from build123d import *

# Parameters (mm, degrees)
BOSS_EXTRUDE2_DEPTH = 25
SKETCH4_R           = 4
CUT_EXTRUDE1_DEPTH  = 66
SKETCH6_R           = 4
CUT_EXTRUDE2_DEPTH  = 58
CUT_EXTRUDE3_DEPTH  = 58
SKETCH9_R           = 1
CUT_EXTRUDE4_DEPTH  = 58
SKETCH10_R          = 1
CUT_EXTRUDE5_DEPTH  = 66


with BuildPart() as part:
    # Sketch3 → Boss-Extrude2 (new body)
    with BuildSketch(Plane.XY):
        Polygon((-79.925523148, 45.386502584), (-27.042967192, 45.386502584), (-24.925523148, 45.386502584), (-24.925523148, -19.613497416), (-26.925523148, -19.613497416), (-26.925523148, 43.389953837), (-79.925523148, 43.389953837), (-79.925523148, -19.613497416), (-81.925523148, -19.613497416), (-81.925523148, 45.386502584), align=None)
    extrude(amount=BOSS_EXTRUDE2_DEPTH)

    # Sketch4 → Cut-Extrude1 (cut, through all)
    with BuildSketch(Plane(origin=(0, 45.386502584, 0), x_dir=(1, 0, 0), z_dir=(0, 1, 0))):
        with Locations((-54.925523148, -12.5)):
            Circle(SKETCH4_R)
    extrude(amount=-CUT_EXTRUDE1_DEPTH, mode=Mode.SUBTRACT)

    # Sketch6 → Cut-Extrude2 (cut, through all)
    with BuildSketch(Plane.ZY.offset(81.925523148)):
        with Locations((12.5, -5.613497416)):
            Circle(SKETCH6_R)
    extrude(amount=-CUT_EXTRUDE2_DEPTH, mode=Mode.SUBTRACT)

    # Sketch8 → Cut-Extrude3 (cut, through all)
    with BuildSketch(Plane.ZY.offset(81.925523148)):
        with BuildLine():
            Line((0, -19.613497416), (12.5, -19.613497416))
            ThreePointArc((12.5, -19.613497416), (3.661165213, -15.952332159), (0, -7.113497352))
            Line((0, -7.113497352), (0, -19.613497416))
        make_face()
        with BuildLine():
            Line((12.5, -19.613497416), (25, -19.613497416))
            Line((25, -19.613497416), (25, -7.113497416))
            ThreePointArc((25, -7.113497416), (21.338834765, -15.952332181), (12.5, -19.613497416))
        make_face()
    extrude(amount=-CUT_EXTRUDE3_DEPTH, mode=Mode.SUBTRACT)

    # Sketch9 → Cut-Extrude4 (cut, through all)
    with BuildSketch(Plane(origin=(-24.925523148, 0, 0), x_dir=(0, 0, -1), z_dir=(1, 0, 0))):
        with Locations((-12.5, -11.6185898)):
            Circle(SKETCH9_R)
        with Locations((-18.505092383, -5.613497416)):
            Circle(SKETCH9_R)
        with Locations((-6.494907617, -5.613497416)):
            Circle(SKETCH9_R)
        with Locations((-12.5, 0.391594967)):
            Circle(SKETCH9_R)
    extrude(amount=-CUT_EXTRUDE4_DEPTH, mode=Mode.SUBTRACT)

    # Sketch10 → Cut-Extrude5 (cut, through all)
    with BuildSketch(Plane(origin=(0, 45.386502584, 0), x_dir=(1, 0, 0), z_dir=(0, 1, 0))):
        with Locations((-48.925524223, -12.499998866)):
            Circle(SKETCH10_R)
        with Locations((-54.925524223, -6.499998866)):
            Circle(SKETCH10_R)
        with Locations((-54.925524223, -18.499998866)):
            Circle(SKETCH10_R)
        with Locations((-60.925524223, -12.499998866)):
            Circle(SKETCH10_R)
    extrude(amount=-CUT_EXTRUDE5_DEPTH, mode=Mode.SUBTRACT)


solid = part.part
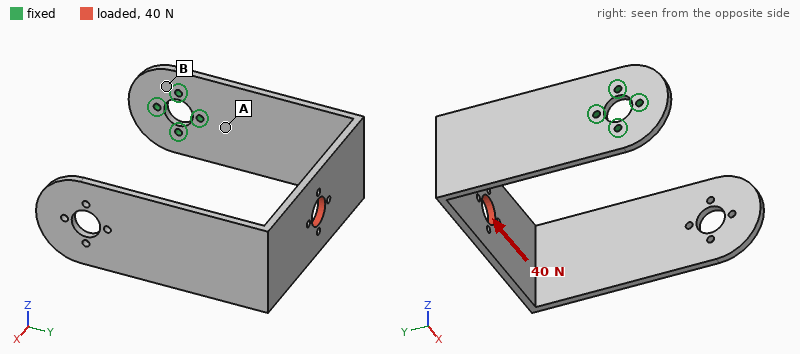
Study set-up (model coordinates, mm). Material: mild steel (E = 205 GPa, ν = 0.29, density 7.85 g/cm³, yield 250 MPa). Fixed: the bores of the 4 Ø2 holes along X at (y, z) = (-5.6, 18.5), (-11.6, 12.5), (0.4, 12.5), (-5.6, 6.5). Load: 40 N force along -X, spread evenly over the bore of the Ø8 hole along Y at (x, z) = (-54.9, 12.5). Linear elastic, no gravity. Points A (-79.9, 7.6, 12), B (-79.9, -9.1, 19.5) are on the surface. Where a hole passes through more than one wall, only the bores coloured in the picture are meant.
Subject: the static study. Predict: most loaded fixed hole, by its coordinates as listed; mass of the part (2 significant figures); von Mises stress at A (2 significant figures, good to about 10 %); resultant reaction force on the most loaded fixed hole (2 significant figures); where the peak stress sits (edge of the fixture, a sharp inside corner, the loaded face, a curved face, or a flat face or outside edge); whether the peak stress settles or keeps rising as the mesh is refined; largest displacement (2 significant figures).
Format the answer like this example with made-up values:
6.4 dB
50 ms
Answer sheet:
(0.4, 12.5)
67 g
80 MPa
180 N
edge of the fixture
keeps rising
0.75 mm
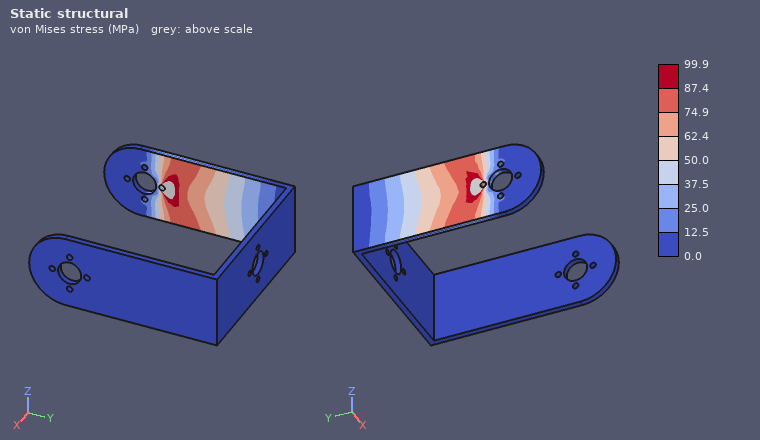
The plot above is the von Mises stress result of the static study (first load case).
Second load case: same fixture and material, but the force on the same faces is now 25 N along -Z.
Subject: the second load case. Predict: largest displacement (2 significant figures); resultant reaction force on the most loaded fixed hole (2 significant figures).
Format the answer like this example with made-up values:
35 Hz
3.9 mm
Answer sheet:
0.32 mm
64 N
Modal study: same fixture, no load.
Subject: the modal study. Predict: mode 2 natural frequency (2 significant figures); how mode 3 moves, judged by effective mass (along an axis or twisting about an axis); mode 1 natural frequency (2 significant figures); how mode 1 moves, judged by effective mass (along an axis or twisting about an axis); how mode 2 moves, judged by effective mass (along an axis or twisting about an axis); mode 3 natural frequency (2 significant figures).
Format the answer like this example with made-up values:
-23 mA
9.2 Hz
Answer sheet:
160 Hz
along X
110 Hz
along Y
along Z
250 Hz
